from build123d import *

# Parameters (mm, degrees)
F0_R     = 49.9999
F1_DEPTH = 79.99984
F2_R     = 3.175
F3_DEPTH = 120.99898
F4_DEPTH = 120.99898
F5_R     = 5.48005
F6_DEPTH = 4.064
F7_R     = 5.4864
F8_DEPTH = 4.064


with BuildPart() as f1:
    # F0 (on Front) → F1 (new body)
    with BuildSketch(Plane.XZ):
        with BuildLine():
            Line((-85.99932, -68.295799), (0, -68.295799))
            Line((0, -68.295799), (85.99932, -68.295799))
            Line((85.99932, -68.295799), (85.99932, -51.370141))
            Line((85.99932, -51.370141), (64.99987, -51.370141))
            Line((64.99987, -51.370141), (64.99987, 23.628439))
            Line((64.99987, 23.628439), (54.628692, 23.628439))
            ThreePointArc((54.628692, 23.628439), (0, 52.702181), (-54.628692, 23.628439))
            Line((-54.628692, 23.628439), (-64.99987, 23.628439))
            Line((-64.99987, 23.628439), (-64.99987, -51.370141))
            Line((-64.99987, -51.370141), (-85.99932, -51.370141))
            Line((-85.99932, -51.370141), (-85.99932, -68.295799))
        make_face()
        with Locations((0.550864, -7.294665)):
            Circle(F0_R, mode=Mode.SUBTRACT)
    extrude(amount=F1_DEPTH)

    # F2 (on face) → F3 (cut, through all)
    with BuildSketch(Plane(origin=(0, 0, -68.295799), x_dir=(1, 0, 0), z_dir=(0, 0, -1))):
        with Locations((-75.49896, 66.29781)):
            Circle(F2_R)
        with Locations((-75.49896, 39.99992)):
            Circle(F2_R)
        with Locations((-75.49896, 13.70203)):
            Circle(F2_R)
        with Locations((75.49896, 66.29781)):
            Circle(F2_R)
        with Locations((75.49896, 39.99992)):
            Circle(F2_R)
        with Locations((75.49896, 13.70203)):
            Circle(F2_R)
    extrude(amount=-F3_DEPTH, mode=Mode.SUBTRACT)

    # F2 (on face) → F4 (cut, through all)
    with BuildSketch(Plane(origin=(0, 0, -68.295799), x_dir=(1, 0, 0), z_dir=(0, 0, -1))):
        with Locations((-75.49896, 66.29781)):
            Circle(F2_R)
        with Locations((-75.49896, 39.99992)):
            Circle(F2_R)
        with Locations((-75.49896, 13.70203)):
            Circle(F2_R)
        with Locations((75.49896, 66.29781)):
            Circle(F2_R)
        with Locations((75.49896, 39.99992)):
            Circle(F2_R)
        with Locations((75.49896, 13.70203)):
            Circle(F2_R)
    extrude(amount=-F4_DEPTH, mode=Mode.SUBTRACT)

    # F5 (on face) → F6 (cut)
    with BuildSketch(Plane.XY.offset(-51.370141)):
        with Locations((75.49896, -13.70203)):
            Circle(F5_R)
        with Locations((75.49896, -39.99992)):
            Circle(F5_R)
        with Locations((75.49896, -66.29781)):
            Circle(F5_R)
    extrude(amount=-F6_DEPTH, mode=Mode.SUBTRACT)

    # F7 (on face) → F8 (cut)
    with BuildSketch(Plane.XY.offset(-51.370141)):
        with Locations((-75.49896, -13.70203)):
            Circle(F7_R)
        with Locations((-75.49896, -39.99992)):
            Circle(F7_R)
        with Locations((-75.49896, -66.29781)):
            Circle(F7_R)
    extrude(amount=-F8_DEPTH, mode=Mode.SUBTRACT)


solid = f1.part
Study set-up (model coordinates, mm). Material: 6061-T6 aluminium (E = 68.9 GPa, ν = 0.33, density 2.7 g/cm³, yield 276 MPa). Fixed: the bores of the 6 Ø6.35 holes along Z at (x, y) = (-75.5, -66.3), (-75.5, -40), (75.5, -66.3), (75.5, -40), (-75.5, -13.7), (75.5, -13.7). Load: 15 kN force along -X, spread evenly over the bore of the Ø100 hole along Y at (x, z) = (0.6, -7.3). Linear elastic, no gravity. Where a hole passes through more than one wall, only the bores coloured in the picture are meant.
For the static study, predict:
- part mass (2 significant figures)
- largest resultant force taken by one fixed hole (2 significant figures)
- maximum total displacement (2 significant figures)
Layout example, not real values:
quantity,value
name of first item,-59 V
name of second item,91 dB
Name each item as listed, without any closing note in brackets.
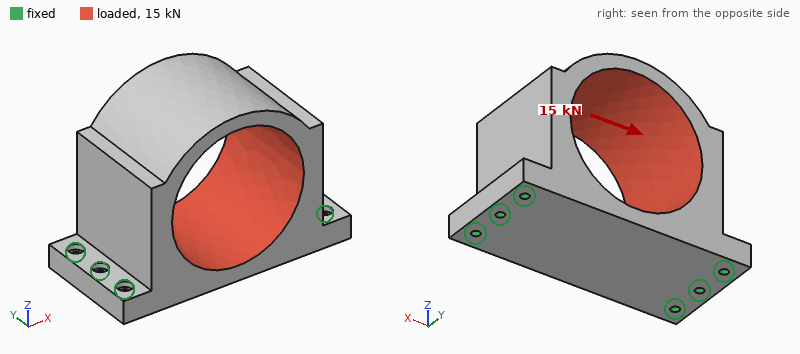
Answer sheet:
quantity,value
part mass,1.5 kg
largest resultant force taken by one fixed hole,3.3 kN
maximum total displacement,0.14 mm
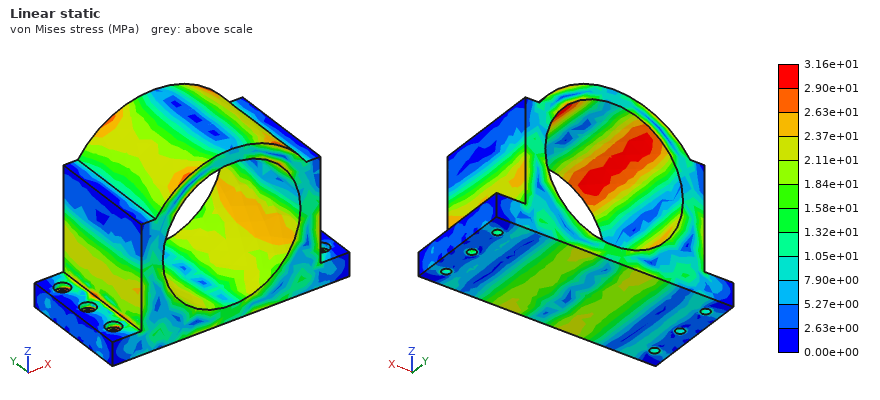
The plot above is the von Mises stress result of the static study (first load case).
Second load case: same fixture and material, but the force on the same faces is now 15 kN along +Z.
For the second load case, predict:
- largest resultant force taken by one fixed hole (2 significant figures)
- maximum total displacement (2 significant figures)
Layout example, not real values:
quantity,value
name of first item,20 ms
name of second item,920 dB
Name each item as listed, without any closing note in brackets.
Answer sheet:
quantity,value
largest resultant force taken by one fixed hole,2.6 kN
maximum total displacement,36 µm
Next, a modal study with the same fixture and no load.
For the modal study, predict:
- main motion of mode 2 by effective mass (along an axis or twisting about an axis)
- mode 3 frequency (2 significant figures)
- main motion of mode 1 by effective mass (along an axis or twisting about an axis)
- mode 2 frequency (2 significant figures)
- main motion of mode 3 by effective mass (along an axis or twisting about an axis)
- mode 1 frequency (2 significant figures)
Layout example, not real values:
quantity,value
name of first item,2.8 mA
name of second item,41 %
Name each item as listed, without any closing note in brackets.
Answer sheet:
quantity,value
main motion of mode 2 by effective mass,along Y
mode 3 frequency,2800 Hz
main motion of mode 1 by effective mass,along X
mode 2 frequency,2000 Hz
main motion of mode 3 by effective mass,along Z
mode 1 frequency,1900 Hz
